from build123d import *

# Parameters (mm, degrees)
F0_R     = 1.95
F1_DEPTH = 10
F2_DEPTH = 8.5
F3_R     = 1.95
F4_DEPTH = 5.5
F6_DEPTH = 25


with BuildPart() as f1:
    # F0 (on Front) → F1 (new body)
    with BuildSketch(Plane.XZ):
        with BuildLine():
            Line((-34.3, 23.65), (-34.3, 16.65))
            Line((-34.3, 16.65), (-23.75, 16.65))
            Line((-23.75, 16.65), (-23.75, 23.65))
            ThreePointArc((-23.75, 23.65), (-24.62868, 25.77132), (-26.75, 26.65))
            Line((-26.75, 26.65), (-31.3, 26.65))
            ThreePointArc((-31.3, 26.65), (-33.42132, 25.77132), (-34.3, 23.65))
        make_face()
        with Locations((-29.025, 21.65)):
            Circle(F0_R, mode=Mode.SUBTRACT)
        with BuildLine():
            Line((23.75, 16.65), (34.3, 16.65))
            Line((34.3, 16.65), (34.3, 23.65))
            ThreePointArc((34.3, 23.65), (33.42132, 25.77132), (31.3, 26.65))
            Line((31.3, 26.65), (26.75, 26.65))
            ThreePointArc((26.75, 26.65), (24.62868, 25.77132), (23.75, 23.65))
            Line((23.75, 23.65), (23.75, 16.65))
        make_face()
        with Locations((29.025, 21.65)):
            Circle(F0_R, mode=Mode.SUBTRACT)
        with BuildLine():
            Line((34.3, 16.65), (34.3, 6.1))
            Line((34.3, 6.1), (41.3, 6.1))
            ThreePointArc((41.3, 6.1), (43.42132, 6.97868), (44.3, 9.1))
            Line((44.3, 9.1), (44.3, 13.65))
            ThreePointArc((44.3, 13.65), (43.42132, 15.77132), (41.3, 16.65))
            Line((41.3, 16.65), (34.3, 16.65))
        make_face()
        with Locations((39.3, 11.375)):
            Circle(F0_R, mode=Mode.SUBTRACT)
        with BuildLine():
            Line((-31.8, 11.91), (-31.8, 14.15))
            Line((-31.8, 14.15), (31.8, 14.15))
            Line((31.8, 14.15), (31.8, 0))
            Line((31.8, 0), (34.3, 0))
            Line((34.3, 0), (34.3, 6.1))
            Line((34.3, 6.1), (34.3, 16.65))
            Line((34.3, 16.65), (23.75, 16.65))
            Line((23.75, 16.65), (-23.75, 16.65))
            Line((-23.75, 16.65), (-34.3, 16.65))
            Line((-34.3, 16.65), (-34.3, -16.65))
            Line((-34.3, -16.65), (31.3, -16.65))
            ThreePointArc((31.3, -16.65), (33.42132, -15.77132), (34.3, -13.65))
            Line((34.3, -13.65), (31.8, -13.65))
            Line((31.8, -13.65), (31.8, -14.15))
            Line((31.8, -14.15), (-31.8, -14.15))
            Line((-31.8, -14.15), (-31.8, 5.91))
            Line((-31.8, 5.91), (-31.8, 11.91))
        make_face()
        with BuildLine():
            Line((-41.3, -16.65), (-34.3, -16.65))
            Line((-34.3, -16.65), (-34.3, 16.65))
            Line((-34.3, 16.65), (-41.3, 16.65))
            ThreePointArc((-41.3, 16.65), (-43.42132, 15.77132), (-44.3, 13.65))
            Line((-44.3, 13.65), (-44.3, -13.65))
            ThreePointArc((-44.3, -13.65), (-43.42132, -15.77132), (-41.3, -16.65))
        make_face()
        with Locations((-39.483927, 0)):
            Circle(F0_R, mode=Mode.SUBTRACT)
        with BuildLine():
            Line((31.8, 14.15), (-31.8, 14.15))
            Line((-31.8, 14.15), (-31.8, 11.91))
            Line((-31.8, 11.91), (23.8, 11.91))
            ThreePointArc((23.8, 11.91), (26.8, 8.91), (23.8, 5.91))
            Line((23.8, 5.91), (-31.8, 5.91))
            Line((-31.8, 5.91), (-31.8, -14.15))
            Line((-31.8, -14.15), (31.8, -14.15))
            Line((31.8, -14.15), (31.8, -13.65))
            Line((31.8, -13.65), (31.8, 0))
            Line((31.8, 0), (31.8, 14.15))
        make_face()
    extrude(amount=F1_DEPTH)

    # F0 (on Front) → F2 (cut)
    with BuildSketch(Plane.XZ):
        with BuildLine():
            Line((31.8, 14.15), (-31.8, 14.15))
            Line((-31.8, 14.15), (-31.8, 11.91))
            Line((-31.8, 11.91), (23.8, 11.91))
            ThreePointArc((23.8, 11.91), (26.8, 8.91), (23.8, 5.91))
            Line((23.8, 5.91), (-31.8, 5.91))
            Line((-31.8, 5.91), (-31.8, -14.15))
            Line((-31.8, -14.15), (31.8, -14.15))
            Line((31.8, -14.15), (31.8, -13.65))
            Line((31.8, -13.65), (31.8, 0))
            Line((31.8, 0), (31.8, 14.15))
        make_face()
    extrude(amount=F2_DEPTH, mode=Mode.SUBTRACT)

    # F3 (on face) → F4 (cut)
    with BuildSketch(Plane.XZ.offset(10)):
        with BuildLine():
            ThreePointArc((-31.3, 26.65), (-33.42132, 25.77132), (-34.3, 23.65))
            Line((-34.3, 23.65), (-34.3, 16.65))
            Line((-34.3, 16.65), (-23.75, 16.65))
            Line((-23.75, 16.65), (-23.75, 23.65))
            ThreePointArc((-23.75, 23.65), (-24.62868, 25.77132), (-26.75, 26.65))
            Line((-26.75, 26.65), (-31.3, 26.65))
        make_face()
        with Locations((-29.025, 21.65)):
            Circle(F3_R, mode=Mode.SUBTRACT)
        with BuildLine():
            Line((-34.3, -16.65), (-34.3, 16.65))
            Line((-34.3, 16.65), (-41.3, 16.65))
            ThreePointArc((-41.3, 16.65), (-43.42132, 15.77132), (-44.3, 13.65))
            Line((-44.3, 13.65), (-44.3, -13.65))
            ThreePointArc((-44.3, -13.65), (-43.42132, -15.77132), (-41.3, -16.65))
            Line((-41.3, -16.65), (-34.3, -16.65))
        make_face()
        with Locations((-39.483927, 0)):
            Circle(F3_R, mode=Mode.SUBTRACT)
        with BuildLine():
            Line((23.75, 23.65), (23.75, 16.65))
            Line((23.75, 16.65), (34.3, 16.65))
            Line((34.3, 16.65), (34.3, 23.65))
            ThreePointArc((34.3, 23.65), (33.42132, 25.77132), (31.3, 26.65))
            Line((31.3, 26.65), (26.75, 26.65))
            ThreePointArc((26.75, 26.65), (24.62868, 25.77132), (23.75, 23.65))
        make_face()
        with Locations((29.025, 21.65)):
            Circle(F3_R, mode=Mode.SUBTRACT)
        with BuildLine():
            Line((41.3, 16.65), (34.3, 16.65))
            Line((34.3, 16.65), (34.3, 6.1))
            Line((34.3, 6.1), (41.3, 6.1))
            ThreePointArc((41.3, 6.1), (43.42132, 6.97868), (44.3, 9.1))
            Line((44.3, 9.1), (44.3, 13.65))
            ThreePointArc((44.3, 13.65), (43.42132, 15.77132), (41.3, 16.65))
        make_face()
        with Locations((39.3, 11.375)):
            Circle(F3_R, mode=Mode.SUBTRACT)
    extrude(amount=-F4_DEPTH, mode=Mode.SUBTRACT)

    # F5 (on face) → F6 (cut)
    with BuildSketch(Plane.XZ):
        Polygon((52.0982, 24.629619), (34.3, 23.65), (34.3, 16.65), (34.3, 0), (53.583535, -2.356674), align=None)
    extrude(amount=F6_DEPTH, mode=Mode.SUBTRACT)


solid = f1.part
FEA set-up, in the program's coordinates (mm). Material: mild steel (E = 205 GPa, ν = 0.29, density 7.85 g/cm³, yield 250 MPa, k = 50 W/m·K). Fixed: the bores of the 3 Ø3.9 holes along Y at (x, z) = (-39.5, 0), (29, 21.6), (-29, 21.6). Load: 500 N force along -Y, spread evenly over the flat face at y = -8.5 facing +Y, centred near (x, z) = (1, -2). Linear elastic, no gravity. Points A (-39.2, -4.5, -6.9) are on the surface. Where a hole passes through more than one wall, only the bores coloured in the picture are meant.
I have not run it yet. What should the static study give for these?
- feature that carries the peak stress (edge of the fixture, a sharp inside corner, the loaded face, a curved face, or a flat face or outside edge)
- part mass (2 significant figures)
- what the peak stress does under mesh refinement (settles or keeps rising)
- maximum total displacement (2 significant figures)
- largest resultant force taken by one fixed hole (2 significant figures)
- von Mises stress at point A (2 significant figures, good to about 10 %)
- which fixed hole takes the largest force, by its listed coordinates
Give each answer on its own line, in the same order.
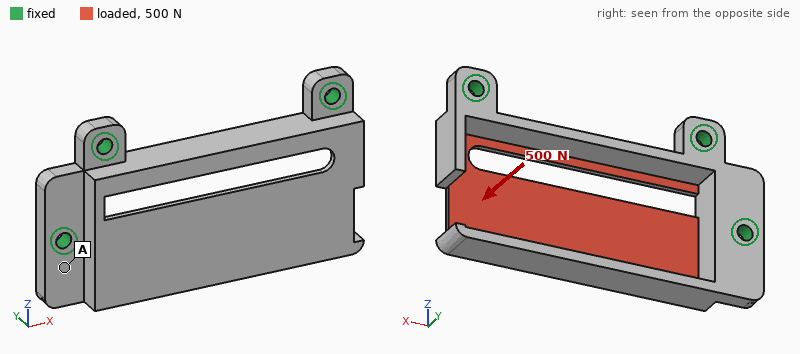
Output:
a sharp inside corner
70 g
keeps rising
0.16 mm
490 N
30 MPa
(-39.5, 0)
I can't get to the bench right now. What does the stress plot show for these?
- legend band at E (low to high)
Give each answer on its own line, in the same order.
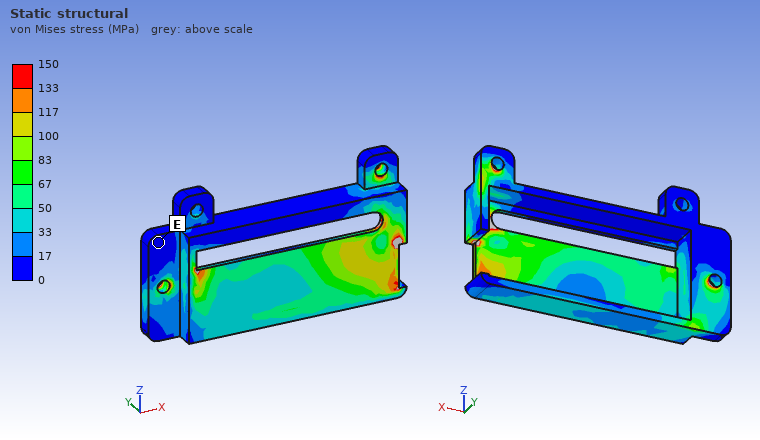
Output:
0 to 17 MPa
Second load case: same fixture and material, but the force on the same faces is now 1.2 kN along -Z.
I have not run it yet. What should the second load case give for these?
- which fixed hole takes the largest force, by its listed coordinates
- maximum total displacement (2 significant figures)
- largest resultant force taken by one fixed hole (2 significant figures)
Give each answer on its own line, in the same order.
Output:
(29, 21.6)
41 µm
610 N
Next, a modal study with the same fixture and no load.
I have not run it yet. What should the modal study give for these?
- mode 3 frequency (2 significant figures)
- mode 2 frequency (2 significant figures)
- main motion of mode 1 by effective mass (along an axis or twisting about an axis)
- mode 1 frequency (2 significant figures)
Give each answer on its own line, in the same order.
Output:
5100 Hz
3000 Hz
along Y
1800 Hz
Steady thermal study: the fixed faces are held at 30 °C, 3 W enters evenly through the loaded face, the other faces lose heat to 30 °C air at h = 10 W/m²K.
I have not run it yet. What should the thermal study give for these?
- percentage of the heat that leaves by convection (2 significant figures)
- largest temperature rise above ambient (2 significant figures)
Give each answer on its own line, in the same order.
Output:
17 %
18 K
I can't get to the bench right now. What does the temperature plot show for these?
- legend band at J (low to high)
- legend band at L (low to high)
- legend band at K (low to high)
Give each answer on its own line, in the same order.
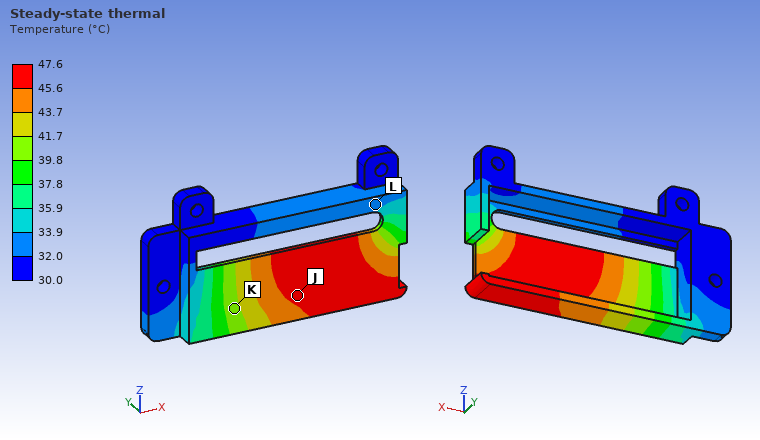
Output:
45.6 to 47.6 °C
32.0 to 33.9 °C
39.8 to 41.7 °C
